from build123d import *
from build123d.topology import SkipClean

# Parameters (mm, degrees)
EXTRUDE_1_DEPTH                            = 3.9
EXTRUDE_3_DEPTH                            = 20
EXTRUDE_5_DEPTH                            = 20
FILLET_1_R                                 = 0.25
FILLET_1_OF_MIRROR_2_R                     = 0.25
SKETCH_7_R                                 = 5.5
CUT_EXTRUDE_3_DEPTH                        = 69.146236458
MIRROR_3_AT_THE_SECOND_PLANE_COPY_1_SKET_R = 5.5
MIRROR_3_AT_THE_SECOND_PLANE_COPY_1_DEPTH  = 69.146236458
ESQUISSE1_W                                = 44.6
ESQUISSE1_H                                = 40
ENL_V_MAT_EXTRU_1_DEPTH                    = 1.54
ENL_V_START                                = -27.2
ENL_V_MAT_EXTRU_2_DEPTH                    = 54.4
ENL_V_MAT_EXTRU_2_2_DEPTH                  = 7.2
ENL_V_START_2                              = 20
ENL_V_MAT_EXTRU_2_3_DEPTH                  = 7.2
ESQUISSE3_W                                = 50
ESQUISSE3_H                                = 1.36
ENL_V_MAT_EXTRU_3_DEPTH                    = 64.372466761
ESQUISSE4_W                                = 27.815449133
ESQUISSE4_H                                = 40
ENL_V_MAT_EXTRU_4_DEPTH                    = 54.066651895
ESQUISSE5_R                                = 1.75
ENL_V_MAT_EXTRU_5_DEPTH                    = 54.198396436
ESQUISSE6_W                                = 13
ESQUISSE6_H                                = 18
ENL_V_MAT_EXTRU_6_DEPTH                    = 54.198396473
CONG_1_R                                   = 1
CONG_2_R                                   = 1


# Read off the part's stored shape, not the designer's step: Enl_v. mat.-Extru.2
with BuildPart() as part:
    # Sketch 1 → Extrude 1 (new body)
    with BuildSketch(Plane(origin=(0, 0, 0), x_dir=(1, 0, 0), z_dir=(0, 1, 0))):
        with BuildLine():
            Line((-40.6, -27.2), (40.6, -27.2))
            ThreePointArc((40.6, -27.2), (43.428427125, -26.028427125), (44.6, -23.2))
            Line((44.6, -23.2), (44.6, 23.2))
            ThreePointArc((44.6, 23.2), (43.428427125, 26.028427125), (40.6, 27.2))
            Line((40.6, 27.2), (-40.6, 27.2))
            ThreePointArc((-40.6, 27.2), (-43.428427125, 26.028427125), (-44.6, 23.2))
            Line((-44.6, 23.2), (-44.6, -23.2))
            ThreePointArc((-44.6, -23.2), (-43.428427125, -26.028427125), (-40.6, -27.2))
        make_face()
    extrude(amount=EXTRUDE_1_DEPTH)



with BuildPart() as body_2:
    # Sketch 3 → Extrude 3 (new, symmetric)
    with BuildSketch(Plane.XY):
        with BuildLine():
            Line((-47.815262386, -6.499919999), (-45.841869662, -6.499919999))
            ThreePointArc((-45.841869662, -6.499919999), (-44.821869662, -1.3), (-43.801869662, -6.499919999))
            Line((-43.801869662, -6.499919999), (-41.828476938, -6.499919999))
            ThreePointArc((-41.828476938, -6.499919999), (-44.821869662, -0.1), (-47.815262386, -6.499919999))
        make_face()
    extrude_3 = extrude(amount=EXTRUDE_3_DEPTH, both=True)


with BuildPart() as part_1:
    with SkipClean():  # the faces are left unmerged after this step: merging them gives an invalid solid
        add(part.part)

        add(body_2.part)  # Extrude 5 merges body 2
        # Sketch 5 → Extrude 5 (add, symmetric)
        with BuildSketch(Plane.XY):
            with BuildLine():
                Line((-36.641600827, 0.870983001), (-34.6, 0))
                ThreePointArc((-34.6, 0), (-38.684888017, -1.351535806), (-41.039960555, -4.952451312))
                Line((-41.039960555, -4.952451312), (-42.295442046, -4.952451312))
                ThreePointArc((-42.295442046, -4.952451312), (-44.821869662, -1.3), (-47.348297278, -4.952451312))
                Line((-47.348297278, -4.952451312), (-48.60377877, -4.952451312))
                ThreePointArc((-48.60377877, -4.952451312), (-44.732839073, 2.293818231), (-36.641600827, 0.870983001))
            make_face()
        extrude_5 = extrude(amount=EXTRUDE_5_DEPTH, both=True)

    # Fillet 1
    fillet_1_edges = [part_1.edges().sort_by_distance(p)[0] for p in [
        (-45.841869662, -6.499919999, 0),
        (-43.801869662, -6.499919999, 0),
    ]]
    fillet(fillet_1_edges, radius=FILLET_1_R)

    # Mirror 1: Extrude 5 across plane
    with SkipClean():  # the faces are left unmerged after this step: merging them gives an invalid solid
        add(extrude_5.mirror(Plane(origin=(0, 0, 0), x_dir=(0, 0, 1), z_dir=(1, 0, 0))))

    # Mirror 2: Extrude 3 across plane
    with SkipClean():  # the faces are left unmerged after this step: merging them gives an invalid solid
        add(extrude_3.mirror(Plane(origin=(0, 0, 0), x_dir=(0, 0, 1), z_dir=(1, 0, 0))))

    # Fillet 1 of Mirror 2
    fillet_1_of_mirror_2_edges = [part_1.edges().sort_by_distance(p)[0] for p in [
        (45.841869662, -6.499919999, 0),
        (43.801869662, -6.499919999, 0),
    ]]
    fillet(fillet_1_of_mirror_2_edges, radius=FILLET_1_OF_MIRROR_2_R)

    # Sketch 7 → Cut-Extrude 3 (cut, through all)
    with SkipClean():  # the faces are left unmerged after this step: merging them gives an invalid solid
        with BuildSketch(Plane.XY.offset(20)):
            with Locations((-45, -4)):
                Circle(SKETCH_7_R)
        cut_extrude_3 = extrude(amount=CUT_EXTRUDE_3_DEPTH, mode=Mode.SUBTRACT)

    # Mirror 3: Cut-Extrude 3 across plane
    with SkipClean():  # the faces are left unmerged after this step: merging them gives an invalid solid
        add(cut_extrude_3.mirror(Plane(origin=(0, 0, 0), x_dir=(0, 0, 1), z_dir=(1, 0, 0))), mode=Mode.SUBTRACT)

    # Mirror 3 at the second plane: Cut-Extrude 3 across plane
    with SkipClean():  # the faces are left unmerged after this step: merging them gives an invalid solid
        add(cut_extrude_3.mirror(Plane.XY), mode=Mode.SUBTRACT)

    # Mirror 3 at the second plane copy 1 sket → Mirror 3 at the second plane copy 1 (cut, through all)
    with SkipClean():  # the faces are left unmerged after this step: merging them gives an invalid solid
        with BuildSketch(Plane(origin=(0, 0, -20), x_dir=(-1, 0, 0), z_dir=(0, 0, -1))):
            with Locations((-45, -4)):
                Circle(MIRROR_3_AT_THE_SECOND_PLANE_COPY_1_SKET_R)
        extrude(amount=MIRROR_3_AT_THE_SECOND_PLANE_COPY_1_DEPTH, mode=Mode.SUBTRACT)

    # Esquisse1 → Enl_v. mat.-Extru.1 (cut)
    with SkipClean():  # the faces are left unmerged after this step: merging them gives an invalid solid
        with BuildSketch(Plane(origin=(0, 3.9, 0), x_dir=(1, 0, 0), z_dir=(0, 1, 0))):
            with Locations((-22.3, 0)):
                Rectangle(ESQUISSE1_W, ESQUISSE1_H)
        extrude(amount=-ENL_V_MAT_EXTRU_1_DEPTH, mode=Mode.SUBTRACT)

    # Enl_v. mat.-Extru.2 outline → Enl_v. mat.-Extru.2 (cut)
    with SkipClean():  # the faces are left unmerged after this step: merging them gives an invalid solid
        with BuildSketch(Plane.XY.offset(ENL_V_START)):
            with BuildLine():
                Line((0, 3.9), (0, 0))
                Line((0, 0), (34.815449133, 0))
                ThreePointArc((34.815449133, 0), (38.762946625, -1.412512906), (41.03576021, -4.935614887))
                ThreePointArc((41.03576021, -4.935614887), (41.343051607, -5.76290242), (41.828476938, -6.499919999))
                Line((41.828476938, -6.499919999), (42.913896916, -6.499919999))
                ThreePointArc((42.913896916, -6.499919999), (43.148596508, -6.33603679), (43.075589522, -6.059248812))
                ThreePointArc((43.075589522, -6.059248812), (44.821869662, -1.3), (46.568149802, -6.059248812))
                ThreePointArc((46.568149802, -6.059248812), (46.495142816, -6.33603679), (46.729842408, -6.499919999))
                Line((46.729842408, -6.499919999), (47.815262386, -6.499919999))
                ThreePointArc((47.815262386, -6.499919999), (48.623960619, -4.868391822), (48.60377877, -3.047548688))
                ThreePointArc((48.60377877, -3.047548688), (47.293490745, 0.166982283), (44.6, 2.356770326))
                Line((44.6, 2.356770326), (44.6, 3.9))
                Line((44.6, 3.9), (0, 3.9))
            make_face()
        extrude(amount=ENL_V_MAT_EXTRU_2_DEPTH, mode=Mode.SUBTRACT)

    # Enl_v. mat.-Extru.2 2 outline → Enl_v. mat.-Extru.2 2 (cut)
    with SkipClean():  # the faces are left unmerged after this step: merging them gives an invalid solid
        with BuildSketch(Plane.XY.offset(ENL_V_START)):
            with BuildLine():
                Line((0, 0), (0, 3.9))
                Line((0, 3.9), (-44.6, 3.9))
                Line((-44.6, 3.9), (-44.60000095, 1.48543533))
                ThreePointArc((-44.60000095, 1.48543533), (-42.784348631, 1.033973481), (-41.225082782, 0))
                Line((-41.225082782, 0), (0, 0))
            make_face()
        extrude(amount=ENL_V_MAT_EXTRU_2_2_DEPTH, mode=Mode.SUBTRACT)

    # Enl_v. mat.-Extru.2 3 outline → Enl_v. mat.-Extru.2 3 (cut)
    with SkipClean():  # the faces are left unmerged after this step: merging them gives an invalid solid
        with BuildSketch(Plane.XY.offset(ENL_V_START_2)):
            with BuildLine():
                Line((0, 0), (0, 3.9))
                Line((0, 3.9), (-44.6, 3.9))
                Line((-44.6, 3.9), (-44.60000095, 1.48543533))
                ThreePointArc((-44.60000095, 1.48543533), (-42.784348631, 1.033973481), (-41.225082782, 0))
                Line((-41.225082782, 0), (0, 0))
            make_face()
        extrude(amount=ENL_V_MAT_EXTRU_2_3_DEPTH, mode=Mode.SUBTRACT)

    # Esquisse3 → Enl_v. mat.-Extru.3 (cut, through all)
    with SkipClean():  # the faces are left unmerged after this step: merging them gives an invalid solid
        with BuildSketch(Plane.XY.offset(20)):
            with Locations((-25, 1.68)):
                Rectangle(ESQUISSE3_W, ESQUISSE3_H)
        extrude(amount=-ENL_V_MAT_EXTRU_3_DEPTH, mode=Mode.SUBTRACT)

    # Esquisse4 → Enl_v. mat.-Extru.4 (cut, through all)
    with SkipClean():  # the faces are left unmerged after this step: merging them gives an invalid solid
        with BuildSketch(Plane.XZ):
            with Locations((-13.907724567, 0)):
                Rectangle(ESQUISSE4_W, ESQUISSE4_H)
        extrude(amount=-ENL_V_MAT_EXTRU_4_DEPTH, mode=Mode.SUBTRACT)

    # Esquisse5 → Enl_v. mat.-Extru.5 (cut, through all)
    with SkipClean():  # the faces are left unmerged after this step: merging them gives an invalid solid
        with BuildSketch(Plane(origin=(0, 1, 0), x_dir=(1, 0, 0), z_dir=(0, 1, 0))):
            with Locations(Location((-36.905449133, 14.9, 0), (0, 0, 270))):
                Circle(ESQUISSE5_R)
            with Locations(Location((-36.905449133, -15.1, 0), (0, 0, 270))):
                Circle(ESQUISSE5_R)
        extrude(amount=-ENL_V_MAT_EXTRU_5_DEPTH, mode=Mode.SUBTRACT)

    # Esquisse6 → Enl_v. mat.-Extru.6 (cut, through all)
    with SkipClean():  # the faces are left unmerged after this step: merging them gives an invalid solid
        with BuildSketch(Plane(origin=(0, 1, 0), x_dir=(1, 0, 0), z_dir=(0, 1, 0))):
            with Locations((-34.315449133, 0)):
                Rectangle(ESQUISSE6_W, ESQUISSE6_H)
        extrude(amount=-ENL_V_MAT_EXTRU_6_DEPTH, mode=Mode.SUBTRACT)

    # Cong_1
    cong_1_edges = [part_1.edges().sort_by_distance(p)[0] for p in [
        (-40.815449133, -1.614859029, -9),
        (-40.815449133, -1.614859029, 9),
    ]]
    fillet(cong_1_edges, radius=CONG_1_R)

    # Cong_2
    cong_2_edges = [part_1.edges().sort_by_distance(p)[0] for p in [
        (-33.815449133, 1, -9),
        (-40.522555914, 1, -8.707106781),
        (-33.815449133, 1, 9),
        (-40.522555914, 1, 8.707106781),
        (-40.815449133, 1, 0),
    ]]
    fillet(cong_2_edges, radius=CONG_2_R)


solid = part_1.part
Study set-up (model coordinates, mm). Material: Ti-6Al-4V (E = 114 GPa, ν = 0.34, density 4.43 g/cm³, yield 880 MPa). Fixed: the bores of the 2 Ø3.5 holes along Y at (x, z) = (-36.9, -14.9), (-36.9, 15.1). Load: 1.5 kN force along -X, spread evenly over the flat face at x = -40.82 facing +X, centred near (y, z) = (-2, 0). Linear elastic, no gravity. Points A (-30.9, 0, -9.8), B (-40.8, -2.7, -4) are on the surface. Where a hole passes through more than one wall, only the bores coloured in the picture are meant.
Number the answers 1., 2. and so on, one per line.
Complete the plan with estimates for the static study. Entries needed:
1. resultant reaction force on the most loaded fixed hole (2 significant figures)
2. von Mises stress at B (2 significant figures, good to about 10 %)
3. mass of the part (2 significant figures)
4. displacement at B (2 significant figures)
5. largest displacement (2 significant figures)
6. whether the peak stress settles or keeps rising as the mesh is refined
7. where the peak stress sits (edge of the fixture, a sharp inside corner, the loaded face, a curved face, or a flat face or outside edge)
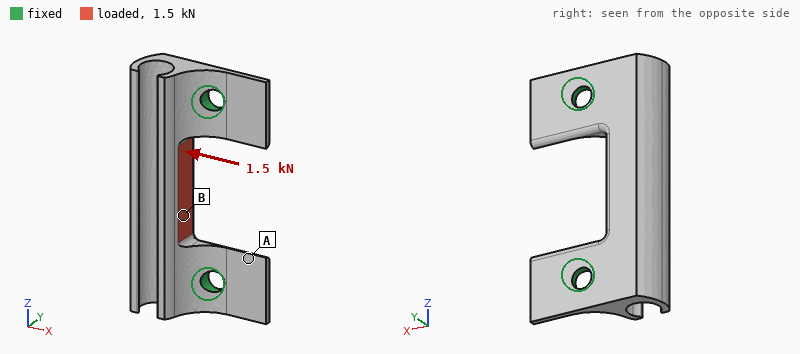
1. 990 N
2. 72 MPa
3. 7.3 g
4. 34 µm
5. 72 µm
6. keeps rising
7. edge of the fixture
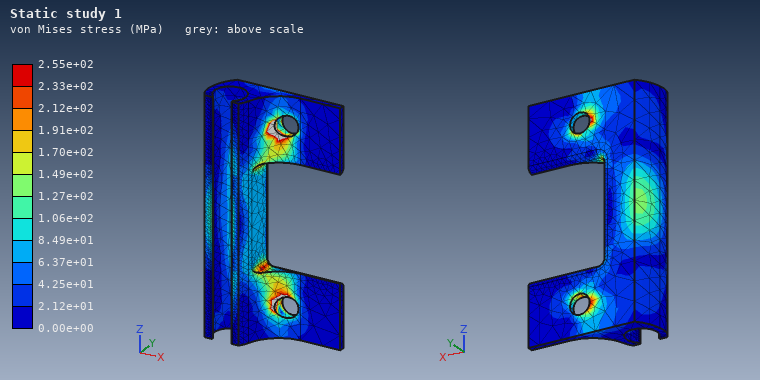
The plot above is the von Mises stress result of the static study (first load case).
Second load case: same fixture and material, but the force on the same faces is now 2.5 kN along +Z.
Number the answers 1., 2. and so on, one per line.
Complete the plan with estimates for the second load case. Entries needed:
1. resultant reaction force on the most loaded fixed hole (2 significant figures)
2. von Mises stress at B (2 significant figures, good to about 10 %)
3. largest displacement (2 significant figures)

1. 1.3 kN
2. 110 MPa
3. 21 µm
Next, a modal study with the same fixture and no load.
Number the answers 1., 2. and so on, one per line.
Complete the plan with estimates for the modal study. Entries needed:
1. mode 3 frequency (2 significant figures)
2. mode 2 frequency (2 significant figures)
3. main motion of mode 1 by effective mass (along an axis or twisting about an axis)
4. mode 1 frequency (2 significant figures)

1. 13 kHz
2. 13 kHz
3. along Y
4. 8800 Hz
